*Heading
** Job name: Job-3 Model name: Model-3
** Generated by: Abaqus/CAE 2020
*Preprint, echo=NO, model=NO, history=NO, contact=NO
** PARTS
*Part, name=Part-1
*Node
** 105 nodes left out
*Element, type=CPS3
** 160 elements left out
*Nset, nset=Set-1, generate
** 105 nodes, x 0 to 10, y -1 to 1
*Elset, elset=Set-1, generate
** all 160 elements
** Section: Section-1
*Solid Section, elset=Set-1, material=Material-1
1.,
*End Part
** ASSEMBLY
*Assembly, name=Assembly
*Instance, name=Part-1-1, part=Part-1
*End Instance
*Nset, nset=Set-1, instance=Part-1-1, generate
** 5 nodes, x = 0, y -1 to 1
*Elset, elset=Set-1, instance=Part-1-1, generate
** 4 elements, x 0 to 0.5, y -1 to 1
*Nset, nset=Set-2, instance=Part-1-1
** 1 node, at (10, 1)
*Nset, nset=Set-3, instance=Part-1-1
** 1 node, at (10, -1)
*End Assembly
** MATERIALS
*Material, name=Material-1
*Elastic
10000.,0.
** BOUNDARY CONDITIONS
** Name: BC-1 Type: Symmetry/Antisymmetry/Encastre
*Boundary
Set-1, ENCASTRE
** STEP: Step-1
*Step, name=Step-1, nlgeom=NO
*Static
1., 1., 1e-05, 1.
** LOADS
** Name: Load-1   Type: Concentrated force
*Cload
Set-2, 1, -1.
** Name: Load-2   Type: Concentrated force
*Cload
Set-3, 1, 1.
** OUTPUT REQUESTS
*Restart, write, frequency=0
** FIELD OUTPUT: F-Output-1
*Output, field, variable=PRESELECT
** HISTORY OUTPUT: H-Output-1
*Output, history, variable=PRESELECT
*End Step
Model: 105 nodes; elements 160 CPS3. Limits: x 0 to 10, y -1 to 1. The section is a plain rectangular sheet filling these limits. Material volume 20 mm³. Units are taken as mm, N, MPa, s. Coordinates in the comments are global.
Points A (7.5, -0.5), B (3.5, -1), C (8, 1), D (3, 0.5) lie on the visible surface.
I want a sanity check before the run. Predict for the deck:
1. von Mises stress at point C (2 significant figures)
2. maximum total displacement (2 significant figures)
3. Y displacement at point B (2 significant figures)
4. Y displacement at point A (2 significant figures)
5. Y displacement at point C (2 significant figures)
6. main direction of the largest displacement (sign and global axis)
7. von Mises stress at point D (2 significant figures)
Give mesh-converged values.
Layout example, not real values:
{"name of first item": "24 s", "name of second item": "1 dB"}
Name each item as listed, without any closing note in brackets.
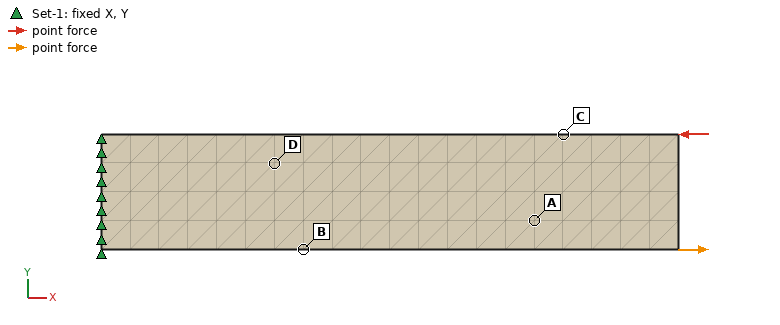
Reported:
{"von Mises stress at point C": "3.0 MPa", "maximum total displacement": "0.016 mm", "Y displacement at point B": "0.0018 mm", "Y displacement at point A": "0.0084 mm", "Y displacement at point C": "0.0096 mm", "main direction of the largest displacement": "+Y", "von Mises stress at point D": "1.5 MPa"}
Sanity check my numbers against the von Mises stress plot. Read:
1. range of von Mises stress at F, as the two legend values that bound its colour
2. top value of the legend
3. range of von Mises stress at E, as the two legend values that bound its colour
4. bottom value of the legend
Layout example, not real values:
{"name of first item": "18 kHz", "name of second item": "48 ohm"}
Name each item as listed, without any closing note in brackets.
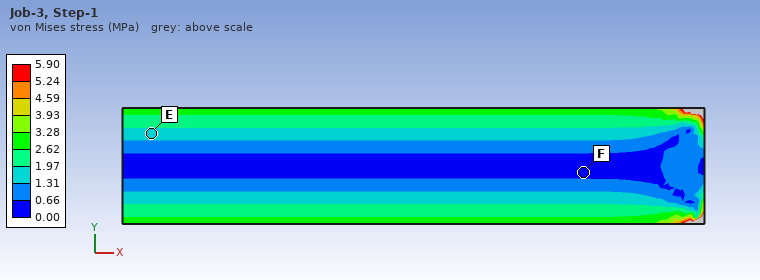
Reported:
{"range of von Mises stress at F, as the two legend values that bound its colour": "0.00 to 0.66 MPa", "top value of the legend": "5.90 MPa", "range of von Mises stress at E, as the two legend values that bound its colour": "1.31 to 1.97 MPa", "bottom value of the legend": "0.00 MPa"}
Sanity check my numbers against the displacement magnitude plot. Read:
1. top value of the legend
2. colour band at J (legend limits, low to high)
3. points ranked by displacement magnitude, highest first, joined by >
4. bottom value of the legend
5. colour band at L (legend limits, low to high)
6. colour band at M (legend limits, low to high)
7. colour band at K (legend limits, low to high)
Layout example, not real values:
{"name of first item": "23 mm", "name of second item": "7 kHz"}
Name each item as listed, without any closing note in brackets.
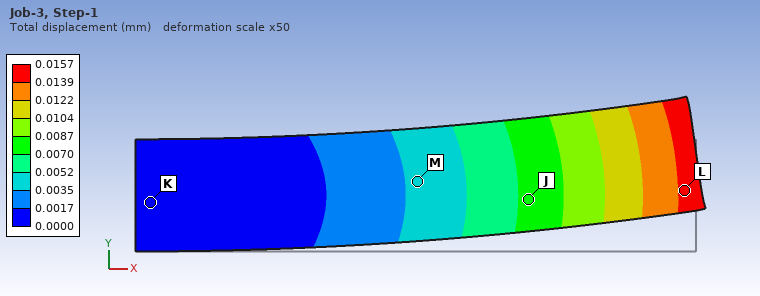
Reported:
{"top value of the legend": "0.0157 mm", "colour band at J": "0.0070 to 0.0087 mm", "points ranked by displacement magnitude, highest first, joined by >": "L > J > M > K", "bottom value of the legend": "0.0000 mm", "colour band at L": "0.0139 to 0.0157 mm", "colour band at M": "0.0035 to 0.0052 mm", "colour band at K": "0.0000 to 0.0017 mm"}
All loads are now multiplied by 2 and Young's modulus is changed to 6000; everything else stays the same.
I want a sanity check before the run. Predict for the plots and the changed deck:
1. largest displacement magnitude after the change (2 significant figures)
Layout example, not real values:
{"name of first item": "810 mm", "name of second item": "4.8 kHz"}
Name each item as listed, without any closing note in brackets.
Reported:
{"largest displacement magnitude after the change": "0.052 mm"}
